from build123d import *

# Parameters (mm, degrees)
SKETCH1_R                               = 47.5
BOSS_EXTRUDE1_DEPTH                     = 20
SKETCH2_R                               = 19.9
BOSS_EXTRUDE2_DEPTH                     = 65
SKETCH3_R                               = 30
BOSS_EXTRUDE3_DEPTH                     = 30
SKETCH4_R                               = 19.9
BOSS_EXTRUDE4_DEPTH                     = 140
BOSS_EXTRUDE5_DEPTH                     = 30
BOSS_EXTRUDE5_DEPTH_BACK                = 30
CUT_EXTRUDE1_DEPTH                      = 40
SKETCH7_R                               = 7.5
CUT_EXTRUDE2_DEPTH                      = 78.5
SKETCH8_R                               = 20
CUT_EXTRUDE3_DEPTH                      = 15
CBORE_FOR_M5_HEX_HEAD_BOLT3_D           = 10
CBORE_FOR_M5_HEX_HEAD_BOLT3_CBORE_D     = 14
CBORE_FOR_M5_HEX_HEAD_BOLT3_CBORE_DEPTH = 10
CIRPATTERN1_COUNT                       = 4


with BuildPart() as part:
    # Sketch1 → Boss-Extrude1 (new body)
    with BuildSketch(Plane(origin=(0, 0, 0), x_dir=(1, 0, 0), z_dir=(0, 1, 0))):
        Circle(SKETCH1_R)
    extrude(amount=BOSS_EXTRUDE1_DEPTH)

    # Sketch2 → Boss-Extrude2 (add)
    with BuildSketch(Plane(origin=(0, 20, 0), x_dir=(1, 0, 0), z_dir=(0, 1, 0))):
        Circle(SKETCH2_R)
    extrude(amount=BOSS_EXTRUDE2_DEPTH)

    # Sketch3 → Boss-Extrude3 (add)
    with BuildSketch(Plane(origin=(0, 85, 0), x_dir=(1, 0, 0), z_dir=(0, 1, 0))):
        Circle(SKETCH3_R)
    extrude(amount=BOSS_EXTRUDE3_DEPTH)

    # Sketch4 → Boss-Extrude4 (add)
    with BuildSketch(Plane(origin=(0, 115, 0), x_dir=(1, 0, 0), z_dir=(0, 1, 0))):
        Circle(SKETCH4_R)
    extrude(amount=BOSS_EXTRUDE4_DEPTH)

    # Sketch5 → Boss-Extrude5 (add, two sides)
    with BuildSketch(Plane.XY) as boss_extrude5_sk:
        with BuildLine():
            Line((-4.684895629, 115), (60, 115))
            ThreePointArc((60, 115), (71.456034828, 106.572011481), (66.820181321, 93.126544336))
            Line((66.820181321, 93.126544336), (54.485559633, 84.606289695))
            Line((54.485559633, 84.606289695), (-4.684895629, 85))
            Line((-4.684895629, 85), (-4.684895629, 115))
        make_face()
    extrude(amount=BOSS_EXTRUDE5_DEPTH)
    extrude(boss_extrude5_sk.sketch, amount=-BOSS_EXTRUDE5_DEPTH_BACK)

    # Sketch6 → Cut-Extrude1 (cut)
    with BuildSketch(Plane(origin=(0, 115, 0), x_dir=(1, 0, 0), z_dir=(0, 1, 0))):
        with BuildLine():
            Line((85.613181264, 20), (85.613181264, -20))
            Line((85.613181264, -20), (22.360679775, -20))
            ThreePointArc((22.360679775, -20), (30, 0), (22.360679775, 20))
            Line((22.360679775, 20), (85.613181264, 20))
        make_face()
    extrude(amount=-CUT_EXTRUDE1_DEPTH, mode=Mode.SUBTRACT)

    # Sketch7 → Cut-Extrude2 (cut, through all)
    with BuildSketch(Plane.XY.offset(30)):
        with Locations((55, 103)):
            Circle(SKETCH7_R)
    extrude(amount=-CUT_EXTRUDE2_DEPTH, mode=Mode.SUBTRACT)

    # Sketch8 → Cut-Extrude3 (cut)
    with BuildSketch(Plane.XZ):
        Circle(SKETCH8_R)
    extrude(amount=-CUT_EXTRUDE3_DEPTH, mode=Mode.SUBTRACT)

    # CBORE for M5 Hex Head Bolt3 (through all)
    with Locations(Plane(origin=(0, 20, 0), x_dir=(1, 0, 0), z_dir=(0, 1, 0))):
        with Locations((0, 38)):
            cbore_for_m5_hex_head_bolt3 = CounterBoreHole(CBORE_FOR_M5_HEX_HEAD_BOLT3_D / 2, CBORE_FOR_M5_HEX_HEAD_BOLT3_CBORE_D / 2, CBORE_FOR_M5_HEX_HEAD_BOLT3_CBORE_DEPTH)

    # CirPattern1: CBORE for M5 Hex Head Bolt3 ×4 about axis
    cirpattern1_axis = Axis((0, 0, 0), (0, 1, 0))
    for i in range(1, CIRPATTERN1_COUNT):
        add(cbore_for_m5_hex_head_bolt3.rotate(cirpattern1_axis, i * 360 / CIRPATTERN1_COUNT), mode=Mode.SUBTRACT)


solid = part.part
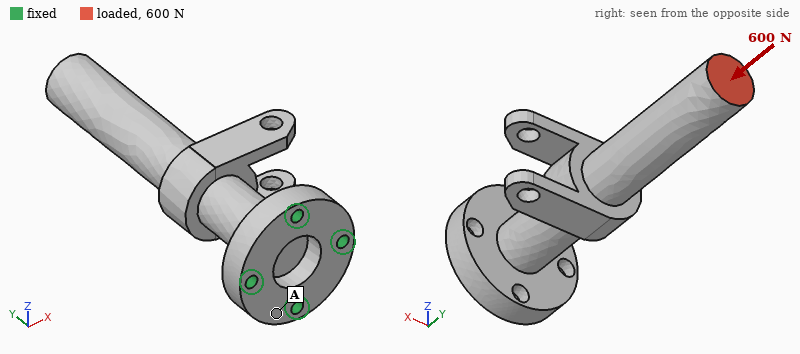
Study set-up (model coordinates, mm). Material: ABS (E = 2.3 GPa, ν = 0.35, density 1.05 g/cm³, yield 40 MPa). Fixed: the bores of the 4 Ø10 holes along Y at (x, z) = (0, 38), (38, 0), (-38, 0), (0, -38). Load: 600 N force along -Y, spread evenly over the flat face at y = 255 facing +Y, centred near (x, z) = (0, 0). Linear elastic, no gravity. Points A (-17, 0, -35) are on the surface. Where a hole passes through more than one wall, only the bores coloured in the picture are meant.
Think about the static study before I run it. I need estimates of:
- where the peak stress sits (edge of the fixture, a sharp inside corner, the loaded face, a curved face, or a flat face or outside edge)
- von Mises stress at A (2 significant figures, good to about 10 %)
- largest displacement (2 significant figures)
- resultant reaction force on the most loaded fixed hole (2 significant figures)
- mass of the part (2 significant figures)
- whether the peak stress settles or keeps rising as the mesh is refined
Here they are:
edge of the fixture
0.29 MPa
63 µm
190 N
510 g
keeps rising
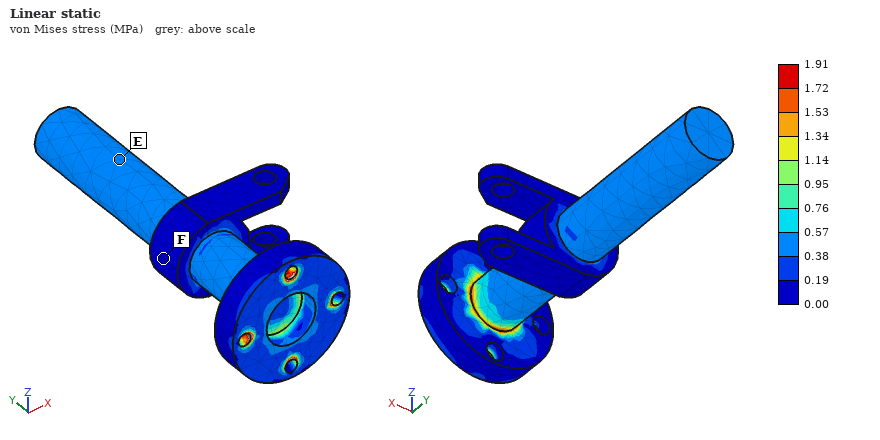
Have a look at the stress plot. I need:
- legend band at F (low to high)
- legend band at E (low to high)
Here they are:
0.00 to 0.19 MPa
0.38 to 0.57 MPa
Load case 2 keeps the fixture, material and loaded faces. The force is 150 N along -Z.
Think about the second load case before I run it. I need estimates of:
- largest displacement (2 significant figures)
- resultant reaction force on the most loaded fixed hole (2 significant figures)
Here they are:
2.9 mm
590 N
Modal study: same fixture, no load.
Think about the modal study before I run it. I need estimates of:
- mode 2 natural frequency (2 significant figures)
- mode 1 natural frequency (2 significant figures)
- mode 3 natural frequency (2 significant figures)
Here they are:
120 Hz
120 Hz
570 Hz
